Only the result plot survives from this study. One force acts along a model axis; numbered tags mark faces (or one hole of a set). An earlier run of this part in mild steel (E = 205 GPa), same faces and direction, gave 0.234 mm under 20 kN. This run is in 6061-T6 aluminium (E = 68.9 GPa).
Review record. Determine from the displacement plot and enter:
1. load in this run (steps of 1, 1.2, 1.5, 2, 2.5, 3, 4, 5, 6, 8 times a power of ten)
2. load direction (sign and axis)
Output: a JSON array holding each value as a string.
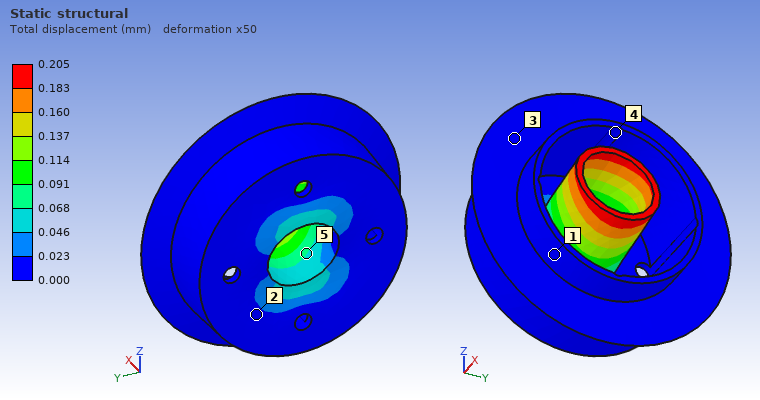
["6 kN", "+Z"]
